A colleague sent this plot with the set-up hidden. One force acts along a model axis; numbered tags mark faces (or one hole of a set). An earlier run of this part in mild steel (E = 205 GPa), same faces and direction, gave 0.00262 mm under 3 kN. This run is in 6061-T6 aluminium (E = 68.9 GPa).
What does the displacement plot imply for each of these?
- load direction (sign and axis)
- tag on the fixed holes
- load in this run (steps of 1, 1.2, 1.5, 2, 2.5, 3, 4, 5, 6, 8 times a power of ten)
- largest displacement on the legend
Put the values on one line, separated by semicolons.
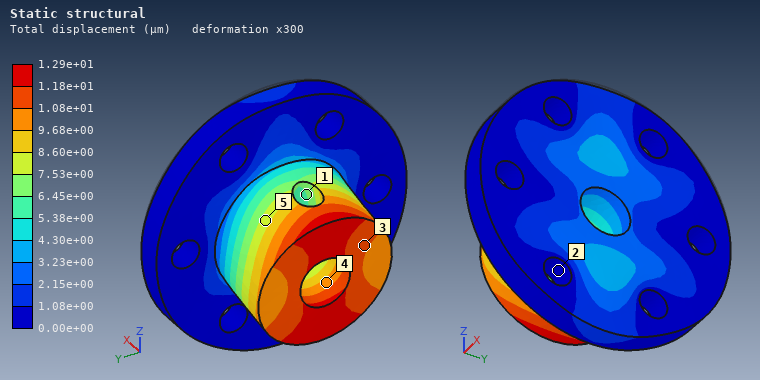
-Z; 2; 5 kN; 1.29e+01 µm
